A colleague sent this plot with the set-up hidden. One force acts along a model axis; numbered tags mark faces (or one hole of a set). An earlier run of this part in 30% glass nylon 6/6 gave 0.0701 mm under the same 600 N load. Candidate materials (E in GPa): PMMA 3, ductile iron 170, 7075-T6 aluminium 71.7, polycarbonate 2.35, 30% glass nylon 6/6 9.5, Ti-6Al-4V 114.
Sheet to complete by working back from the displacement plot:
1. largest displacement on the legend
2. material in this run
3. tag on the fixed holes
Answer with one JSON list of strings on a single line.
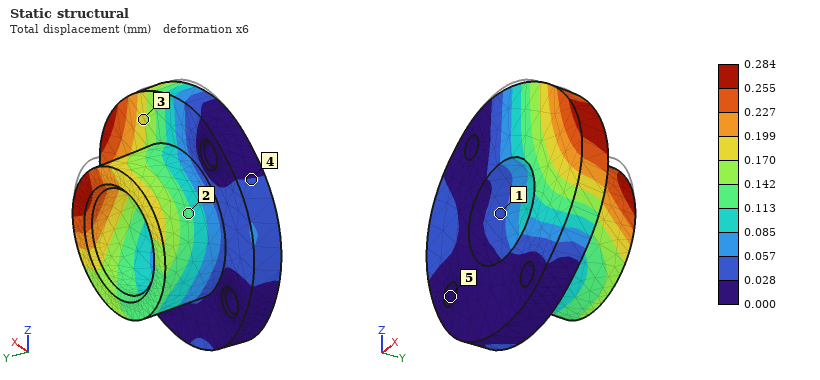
["0.284 mm", "polycarbonate", "5"]
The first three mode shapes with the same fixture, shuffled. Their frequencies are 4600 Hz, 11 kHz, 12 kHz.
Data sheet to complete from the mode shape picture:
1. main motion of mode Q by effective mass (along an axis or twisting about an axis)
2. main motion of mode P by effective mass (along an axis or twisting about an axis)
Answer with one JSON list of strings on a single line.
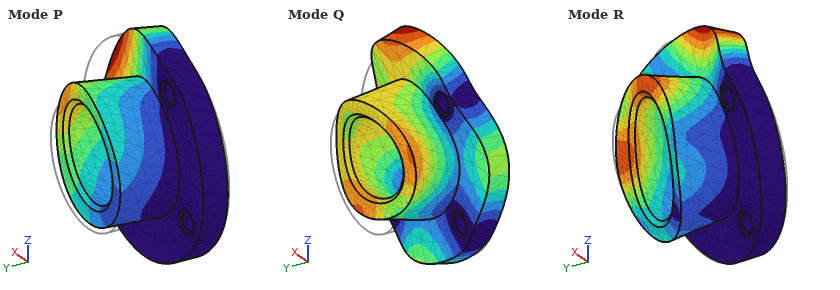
["along Z", "along Y"]
